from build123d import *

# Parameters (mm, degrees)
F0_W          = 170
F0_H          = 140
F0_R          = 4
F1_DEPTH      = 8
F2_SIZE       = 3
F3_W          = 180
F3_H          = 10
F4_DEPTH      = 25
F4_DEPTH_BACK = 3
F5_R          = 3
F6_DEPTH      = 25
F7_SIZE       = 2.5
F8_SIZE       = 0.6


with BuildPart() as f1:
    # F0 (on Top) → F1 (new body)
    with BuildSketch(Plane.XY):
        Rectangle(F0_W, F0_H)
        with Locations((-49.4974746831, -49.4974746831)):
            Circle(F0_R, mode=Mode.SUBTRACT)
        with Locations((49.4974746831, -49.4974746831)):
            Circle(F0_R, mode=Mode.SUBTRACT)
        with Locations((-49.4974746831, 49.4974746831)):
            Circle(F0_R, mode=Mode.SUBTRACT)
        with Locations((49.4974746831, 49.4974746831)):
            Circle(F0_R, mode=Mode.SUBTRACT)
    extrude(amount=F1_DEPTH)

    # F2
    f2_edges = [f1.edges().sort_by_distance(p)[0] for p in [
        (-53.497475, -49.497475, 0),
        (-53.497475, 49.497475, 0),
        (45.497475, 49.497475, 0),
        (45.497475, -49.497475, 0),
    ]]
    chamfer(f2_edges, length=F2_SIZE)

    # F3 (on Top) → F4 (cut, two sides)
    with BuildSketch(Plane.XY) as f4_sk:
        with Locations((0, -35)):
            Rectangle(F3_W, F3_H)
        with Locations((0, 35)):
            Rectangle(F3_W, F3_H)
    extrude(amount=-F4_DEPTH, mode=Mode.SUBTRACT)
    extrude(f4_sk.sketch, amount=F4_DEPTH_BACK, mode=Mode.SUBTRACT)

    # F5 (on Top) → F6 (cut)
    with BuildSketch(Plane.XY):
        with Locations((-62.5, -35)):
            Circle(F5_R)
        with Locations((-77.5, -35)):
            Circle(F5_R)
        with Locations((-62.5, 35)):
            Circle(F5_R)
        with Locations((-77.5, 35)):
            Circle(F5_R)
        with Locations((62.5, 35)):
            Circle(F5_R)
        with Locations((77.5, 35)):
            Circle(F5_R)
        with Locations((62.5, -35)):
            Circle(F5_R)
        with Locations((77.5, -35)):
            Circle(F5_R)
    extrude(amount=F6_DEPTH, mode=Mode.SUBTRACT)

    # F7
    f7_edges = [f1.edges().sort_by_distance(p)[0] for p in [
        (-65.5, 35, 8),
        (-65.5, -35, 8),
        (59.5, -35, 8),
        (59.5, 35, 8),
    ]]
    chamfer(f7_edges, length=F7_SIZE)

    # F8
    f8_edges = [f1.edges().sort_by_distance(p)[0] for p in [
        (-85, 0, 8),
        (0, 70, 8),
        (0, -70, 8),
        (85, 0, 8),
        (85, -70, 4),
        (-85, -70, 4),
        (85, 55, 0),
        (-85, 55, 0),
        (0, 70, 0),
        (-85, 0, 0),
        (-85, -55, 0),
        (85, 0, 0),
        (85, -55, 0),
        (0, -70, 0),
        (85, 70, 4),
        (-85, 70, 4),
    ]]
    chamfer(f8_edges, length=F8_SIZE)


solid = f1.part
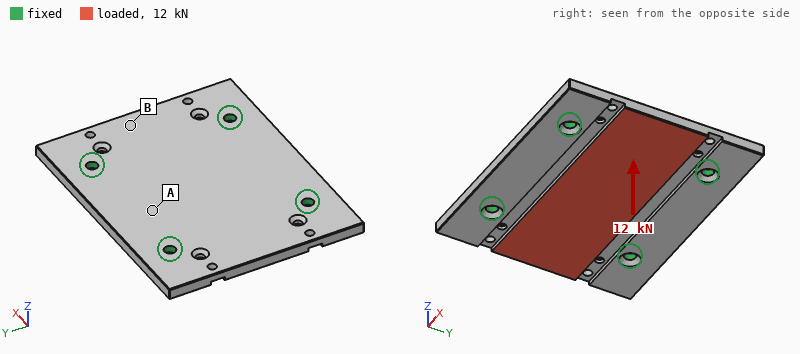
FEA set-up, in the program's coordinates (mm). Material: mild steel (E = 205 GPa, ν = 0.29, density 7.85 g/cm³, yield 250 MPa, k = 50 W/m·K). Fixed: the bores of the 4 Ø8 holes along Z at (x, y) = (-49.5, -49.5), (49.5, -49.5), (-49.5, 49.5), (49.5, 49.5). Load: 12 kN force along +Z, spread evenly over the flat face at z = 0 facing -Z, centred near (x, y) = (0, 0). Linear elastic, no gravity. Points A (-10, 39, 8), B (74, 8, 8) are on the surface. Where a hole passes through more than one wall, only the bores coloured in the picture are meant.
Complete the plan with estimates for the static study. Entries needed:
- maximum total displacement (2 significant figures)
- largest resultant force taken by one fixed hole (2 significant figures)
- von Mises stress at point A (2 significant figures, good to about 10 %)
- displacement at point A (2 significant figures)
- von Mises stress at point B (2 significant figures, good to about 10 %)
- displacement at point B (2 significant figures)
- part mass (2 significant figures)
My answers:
79 µm
3.6 kN
22 MPa
38 µm
54 MPa
69 µm
1.4 kg
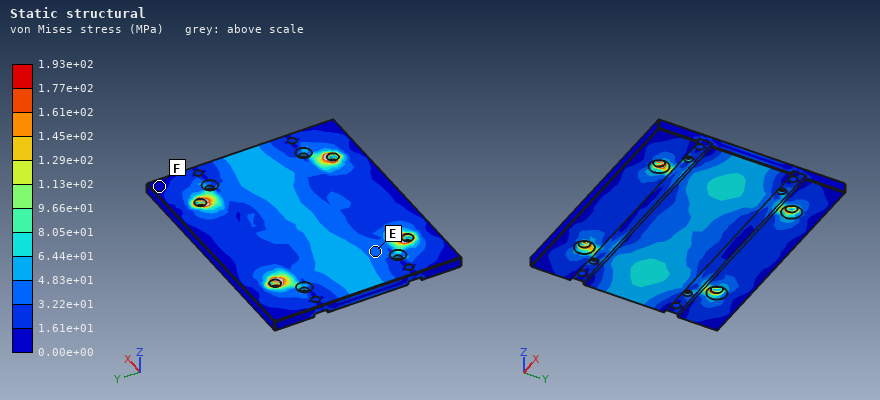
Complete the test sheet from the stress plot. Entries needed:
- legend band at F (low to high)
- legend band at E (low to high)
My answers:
0.00e+00 to 1.61e+01 MPa
3.22e+01 to 4.83e+01 MPa
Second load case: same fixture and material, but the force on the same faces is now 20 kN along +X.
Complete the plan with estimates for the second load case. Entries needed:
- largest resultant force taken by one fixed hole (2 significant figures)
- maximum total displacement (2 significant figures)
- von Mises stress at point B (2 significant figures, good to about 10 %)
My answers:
5.1 kN
33 µm
21 MPa
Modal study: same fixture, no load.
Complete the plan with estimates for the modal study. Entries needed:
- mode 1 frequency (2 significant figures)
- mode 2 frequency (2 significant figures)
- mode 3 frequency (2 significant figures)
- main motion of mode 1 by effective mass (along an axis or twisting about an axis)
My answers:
2600 Hz
2700 Hz
2700 Hz
along Z
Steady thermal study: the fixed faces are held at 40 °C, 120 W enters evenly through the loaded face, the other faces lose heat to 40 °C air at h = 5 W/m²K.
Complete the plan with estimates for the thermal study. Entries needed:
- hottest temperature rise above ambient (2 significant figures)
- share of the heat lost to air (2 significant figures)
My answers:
60 K
5.7 %
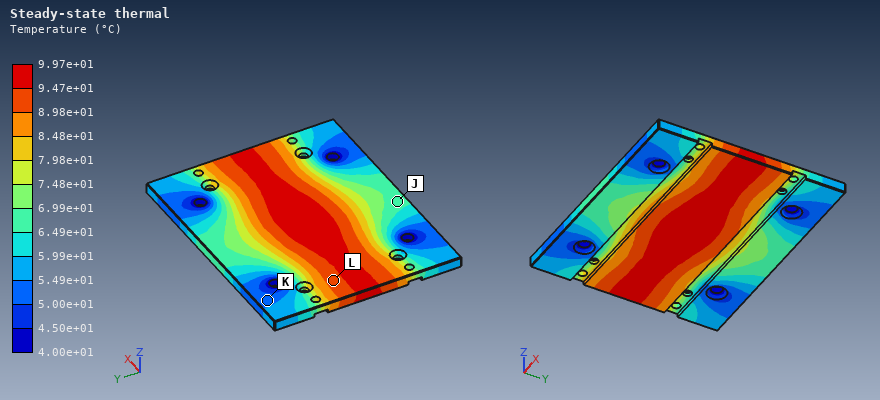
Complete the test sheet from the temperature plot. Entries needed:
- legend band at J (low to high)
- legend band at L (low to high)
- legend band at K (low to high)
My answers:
6.49e+01 to 6.99e+01 °C
8.98e+01 to 9.47e+01 °C
5.00e+01 to 5.49e+01 °C
